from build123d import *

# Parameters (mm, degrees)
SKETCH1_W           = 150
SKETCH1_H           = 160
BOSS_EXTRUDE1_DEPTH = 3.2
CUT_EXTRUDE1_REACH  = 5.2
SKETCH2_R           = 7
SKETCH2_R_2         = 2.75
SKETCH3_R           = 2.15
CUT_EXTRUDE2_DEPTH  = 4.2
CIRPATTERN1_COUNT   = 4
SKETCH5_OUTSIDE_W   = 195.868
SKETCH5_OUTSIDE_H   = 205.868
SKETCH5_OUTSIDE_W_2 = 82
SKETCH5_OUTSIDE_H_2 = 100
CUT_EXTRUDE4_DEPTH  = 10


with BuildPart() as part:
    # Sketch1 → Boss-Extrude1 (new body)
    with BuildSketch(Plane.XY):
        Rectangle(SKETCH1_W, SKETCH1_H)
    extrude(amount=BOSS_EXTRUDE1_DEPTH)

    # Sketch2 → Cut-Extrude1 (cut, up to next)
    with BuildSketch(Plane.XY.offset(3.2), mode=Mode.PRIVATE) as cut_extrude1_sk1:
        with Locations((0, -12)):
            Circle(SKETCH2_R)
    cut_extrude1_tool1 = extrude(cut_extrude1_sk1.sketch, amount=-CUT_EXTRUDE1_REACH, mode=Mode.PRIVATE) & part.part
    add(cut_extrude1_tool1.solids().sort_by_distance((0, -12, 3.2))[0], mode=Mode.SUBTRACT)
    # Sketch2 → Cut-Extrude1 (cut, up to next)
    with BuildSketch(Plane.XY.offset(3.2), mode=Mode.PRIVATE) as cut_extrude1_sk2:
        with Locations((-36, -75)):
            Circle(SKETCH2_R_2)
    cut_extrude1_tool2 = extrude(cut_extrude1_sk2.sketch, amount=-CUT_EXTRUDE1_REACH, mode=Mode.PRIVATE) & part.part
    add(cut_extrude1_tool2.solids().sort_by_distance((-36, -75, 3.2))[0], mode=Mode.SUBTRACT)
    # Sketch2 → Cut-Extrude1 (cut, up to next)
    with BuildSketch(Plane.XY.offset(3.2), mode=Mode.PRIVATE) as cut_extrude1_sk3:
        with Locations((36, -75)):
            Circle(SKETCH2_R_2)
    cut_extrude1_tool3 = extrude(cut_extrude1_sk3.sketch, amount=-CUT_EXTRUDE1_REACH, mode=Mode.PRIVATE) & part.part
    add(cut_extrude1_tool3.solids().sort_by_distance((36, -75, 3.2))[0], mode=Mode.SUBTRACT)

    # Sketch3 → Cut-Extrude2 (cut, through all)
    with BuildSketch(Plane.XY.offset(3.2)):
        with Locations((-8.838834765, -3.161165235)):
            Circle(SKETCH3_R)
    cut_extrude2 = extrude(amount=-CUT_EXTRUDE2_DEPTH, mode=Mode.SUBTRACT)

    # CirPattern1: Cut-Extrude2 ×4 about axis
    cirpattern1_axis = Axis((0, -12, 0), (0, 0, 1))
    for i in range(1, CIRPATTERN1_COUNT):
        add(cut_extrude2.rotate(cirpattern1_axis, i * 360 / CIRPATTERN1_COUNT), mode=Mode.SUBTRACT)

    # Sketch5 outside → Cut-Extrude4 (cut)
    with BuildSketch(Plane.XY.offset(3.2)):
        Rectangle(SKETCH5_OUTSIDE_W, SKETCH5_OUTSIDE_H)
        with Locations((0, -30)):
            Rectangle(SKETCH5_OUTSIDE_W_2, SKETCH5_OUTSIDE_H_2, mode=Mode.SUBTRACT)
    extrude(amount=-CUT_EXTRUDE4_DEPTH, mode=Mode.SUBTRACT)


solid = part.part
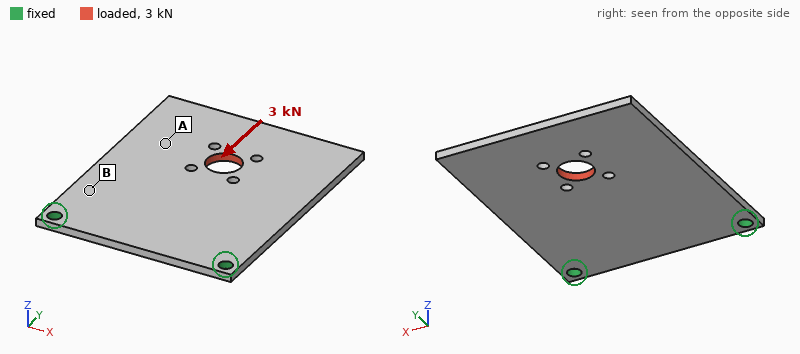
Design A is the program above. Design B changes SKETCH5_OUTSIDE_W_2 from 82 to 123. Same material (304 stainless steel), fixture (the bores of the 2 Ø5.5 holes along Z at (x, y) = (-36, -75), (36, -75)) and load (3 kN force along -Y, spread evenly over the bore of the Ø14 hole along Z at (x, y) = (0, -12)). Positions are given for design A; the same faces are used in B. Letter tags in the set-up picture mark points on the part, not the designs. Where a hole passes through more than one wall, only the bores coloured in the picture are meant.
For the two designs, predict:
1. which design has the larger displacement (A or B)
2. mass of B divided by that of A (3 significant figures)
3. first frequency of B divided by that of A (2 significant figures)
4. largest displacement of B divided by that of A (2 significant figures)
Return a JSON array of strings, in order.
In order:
["A", "1.52", "1.0", "0.90"]
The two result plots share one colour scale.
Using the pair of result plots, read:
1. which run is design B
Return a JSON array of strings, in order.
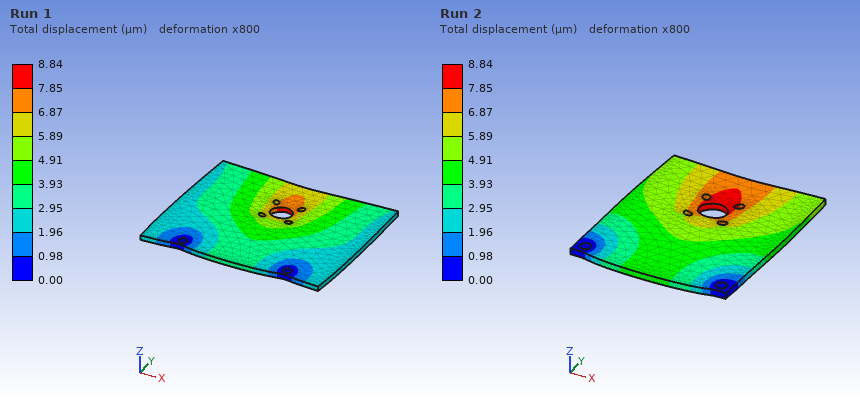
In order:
["Run 1"]
